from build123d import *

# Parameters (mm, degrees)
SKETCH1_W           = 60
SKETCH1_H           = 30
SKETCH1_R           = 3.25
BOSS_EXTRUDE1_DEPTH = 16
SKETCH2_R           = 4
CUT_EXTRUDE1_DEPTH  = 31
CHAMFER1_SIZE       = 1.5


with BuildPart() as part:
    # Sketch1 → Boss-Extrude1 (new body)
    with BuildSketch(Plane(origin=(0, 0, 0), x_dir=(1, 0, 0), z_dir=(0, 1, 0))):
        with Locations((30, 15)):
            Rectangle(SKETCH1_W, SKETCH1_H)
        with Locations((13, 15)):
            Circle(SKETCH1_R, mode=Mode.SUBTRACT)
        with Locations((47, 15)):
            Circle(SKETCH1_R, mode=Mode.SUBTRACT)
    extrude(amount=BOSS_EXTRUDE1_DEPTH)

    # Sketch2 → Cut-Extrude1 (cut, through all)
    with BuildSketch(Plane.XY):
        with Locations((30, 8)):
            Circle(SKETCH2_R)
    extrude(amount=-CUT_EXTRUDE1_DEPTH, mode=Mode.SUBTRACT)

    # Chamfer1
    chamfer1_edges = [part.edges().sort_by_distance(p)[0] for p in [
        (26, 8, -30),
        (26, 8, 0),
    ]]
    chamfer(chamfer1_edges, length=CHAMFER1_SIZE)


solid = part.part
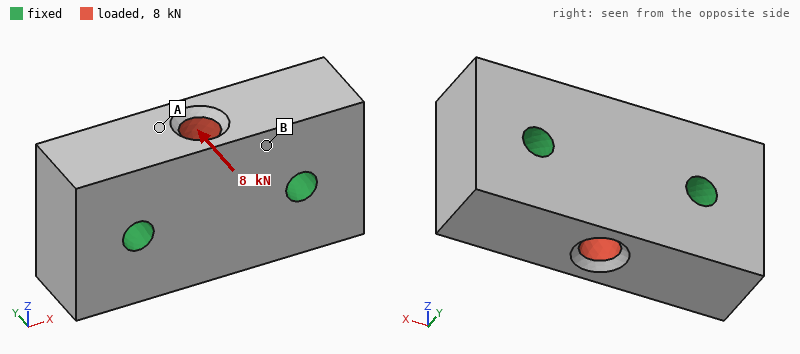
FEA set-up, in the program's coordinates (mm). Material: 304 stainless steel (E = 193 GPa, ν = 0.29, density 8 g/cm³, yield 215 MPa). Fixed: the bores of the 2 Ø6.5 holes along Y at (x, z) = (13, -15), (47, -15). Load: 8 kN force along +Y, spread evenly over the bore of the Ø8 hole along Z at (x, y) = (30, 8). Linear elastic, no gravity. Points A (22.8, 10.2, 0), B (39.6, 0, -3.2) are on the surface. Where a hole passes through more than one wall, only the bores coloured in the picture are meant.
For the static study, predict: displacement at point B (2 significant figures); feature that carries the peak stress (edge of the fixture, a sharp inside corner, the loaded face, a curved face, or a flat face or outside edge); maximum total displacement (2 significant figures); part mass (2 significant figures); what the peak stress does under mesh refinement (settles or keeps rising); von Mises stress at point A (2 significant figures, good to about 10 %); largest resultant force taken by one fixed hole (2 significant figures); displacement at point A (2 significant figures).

2.0 µm
edge of the fixture
3.4 µm
210 g
keeps rising
14 MPa
4.0 kN
2.4 µm
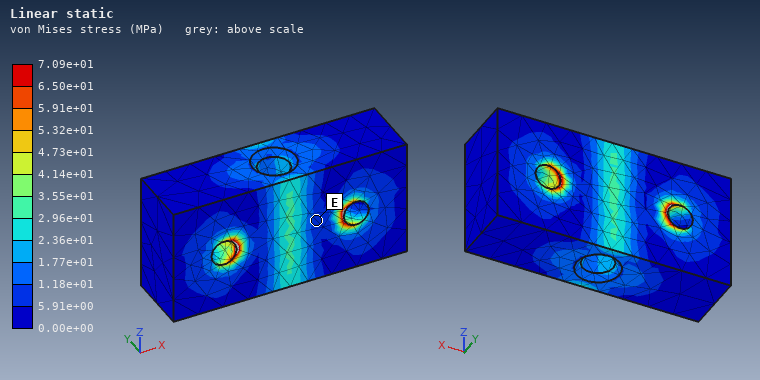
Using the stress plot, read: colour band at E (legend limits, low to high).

5.91e+00 to 1.18e+01 MPa
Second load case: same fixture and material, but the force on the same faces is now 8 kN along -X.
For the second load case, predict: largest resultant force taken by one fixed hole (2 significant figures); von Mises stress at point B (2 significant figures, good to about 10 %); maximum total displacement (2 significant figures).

4.0 kN
3.6 MPa
1.1 µm
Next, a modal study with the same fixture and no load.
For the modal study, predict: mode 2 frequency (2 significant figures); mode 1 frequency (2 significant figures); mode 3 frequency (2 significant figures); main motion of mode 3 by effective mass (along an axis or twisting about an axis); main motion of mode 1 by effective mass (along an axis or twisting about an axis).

29 kHz
28 kHz
32 kHz
twisting about Y
twisting about X
